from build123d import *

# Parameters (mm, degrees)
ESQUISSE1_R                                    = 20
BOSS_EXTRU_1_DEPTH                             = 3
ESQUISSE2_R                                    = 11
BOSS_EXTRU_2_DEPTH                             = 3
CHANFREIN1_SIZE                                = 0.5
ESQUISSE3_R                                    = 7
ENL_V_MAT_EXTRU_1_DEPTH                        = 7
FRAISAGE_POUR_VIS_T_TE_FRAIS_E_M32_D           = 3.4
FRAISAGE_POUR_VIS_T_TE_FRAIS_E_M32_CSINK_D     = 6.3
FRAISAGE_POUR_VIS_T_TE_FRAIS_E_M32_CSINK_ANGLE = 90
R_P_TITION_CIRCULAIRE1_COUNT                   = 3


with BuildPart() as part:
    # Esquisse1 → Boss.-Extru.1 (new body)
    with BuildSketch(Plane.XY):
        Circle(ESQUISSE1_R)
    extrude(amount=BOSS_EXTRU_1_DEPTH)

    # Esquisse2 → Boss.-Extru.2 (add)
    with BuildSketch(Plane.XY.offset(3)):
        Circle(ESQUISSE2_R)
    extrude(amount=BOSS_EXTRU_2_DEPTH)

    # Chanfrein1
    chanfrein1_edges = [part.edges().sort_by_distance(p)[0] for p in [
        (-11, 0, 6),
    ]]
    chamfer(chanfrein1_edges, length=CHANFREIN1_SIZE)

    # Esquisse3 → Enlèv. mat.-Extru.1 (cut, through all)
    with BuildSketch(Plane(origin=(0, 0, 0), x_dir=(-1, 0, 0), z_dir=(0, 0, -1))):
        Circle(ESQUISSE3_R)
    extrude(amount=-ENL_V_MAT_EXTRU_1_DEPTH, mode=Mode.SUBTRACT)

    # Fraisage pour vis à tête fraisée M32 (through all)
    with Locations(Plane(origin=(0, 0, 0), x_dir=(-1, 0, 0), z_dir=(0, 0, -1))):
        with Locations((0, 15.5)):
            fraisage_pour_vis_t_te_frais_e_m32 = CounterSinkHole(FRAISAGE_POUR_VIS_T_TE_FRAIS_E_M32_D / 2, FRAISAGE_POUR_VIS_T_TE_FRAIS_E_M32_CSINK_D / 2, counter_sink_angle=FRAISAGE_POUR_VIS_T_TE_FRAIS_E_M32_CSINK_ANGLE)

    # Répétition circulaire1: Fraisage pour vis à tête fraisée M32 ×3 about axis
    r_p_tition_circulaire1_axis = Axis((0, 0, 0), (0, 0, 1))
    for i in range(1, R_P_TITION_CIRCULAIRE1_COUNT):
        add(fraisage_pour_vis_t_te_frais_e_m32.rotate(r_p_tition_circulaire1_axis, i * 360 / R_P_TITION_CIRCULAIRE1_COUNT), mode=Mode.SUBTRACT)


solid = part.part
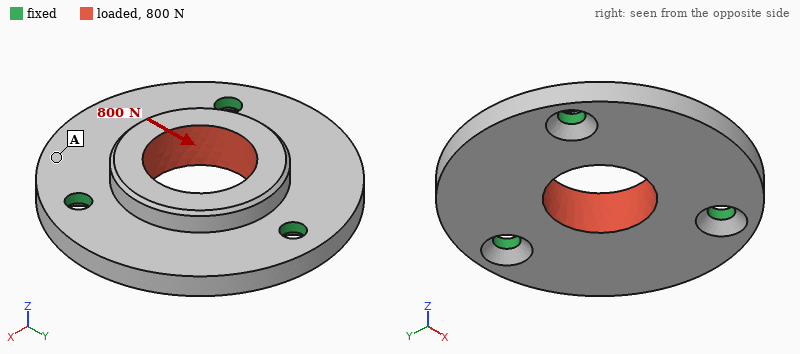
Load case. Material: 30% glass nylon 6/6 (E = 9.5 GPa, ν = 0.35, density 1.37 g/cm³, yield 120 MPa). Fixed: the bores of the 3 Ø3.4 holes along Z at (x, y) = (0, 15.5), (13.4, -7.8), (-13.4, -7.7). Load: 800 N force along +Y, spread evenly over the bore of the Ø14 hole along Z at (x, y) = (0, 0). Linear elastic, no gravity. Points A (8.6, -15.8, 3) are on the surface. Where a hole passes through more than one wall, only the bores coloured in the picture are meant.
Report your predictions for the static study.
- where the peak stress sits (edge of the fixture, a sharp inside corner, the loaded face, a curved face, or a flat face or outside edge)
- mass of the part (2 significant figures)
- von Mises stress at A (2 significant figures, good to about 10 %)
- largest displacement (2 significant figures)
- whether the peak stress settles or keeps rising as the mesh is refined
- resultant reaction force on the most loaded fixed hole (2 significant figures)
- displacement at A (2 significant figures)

edge of the fixture
5.3 g
4.7 MPa
23 µm
keeps rising
280 N
11 µm
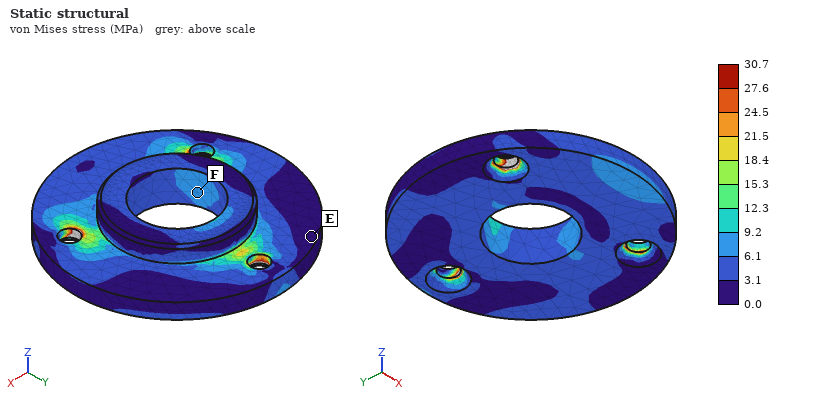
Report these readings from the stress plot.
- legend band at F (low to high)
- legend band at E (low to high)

6.1 to 9.2 MPa
0.0 to 3.1 MPa
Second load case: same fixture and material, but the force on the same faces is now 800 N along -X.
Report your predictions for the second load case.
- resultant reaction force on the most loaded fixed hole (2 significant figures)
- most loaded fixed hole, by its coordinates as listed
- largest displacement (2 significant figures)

290 N
(0, 15.5)
21 µm
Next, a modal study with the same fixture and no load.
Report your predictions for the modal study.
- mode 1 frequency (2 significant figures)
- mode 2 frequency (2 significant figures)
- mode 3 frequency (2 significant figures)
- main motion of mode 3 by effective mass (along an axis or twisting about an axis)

6200 Hz
6200 Hz
7900 Hz
along Z
